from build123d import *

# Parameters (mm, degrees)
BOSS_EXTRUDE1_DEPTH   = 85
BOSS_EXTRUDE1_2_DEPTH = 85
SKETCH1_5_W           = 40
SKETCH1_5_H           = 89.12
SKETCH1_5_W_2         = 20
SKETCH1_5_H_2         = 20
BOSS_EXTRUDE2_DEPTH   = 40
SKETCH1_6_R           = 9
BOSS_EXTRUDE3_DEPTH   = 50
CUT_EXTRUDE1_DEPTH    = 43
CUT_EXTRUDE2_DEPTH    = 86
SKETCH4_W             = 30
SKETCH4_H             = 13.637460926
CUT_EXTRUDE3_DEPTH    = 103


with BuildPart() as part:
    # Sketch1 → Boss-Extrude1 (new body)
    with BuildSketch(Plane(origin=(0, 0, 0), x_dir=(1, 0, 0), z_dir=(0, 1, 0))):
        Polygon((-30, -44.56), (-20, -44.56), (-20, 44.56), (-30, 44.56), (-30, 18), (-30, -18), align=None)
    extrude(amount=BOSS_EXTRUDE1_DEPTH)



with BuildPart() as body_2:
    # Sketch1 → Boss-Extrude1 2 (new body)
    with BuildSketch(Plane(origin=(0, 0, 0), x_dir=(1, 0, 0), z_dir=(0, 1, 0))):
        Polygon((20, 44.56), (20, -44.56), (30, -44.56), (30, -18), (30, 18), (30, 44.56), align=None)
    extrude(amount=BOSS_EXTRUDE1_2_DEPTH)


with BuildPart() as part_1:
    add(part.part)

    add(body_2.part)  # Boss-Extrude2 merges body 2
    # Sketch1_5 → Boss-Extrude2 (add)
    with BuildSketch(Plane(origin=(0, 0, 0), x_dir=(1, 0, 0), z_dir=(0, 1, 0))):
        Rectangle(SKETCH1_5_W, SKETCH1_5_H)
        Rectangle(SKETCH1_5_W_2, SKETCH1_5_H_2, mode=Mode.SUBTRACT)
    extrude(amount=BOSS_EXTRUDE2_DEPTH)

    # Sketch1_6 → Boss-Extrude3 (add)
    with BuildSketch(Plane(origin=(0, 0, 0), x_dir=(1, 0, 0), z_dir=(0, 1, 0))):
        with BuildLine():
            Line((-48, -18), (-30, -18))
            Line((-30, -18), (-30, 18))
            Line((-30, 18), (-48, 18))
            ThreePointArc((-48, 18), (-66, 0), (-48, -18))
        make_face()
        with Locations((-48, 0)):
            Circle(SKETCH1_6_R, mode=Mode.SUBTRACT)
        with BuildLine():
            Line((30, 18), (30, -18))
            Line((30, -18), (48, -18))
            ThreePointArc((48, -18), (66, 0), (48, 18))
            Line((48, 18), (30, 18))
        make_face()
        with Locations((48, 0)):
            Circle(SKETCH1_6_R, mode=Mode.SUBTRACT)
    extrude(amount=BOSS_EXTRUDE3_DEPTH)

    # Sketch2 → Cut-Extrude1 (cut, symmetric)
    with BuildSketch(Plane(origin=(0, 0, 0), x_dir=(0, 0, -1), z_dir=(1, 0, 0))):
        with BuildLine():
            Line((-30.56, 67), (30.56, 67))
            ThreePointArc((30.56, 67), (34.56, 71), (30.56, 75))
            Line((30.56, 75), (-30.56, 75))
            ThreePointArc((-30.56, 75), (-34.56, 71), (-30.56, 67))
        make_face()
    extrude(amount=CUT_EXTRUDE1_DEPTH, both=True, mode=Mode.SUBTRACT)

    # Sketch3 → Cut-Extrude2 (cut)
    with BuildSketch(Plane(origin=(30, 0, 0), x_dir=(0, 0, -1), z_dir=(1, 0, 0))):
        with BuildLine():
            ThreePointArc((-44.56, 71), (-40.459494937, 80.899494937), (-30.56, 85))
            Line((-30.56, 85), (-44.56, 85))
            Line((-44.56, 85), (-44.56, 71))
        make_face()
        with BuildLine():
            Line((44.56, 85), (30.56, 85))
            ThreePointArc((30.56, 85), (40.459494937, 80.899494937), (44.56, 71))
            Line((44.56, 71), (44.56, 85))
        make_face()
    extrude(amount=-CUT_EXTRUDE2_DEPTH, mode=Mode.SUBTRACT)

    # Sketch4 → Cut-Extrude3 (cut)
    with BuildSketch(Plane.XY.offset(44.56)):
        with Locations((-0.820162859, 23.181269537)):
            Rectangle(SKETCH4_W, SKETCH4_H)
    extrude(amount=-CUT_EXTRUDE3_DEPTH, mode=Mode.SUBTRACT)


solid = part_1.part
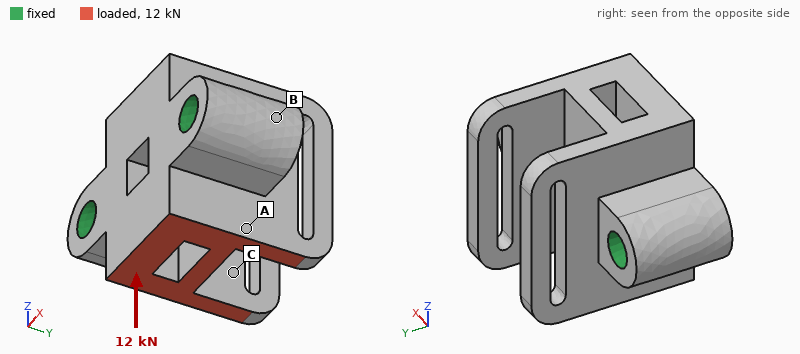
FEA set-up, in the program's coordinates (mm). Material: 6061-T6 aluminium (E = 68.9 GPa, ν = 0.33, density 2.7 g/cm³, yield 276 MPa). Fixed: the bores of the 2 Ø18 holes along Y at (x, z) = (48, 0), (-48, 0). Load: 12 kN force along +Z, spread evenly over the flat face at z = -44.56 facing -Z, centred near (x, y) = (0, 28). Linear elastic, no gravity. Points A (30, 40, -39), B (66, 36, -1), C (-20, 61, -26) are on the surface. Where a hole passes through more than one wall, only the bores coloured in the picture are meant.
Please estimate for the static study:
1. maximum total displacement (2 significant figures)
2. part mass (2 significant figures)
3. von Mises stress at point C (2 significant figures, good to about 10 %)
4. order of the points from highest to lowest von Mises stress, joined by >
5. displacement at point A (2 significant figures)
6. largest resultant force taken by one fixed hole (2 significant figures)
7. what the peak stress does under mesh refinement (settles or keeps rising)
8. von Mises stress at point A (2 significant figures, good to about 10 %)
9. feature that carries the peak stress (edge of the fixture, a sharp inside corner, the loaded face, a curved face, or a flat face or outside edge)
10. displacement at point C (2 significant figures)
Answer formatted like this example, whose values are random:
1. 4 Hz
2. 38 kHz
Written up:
1. 8.5 µm
2. 880 g
3. 4.0 MPa
4. A > C > B
5. 6.0 µm
6. 6.1 kN
7. keeps rising
8. 6.1 MPa
9. edge of the fixture
10. 6.5 µm
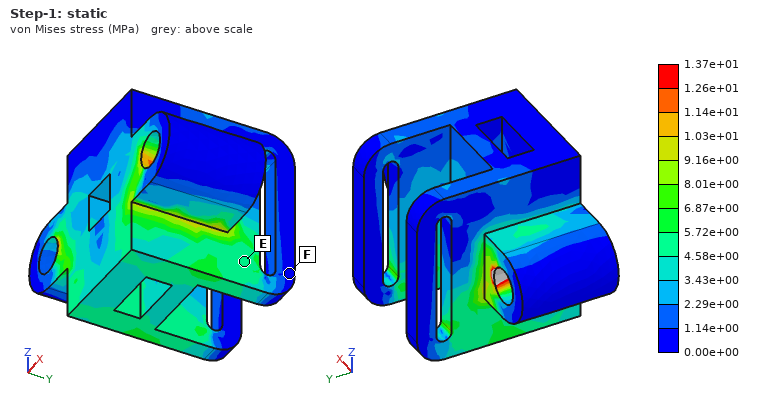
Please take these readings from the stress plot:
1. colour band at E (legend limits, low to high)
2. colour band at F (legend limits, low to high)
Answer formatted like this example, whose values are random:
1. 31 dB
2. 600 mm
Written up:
1. 4.58e+00 to 5.72e+00 MPa
2. 0.00e+00 to 1.14e+00 MPa
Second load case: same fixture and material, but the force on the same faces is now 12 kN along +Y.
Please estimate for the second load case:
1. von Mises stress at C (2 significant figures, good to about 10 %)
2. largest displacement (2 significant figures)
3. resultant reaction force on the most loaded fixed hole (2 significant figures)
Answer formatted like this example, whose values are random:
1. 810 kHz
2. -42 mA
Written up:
1. 6.2 MPa
2. 41 µm
3. 6.1 kN
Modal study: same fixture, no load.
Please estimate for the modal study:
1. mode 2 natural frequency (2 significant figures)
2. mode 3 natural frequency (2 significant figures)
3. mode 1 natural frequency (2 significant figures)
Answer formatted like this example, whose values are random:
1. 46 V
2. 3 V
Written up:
1. 3200 Hz
2. 5200 Hz
3. 3200 Hz
